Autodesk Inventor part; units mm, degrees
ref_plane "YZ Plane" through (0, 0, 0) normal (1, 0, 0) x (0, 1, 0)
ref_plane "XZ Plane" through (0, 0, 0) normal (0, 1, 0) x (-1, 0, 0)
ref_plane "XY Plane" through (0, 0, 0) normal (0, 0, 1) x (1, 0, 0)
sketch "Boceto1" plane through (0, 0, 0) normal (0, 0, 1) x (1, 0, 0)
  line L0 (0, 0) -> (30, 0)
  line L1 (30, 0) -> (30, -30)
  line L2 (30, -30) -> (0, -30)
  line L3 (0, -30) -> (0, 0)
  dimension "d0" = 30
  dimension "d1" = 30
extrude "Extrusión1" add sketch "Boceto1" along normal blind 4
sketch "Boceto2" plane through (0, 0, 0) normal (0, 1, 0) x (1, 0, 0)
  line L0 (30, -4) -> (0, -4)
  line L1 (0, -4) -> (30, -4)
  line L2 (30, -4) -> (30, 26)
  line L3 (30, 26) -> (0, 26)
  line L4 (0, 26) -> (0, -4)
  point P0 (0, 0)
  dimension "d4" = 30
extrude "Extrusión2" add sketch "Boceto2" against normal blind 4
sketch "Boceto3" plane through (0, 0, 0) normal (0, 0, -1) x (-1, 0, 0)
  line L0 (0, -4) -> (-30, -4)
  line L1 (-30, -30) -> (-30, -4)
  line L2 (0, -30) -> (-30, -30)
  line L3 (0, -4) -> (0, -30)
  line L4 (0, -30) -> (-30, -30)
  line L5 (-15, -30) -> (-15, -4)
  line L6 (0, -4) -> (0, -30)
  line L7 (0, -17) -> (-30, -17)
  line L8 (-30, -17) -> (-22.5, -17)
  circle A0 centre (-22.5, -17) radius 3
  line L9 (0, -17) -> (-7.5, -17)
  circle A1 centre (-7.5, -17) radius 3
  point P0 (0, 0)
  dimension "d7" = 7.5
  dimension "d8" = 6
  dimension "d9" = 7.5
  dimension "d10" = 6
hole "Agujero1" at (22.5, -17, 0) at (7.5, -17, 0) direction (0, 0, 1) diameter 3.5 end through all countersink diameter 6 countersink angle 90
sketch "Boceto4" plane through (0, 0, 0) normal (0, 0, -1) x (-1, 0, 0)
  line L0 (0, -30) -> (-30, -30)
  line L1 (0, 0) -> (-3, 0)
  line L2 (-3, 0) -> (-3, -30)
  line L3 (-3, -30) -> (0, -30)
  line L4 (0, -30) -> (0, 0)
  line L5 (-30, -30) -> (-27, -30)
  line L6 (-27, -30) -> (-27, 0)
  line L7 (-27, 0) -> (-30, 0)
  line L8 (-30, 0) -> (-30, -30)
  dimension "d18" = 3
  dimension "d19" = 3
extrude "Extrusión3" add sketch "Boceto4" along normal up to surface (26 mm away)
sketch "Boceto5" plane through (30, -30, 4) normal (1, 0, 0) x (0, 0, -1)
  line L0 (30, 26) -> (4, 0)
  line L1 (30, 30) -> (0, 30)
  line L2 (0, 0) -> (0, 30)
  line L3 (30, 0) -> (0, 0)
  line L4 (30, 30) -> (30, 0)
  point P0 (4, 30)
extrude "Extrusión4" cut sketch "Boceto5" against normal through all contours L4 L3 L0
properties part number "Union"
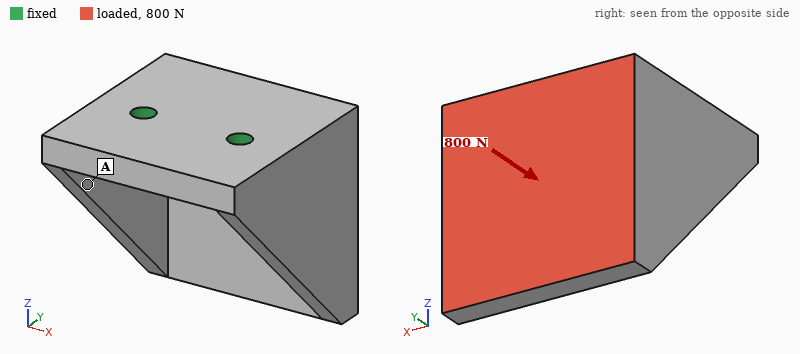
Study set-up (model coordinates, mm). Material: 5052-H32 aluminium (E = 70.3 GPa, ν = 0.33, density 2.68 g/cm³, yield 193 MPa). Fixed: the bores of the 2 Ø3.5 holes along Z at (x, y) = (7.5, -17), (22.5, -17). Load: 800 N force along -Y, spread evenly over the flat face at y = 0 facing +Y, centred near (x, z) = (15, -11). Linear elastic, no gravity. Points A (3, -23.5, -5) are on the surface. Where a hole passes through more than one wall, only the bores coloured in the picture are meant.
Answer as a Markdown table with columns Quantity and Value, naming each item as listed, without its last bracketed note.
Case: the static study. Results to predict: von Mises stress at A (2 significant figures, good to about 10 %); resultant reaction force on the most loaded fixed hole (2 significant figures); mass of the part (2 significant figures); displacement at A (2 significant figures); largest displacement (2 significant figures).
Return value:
| Quantity | Value |
|---|---|
| von Mises stress at A | 25 MPa |
| resultant reaction force on the most loaded fixed hole | 400 N |
| mass of the part | 23 g |
| displacement at A | 0.038 mm |
| largest displacement | 0.14 mm |
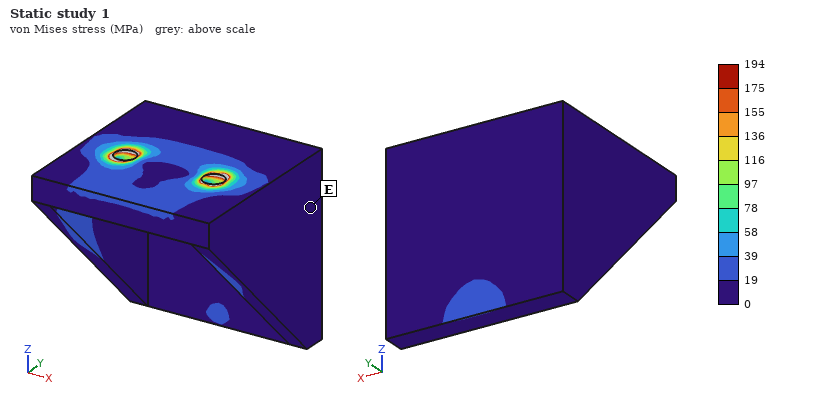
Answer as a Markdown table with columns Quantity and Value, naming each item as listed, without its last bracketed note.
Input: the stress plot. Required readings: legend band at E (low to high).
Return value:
| Quantity | Value |
|---|---|
| legend band at E | 0 to 19 MPa |
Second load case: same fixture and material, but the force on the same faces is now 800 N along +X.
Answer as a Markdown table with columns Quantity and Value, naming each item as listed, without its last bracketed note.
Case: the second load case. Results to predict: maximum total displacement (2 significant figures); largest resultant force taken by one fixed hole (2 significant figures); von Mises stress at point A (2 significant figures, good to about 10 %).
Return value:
| Quantity | Value |
|---|---|
| maximum total displacement | 80 µm |
| largest resultant force taken by one fixed hole | 1.0 kN |
| von Mises stress at point A | 24 MPa |
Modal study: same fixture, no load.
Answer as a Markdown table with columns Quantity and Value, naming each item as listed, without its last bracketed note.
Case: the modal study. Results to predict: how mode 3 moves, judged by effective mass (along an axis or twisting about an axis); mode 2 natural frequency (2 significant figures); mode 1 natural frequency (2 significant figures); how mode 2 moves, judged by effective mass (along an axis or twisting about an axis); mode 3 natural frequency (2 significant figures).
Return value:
| Quantity | Value |
|---|---|
| how mode 3 moves, judged by effective mass | along X |
| mode 2 natural frequency | 4600 Hz |
| mode 1 natural frequency | 3400 Hz |
| how mode 2 moves, judged by effective mass | along X |
| mode 3 natural frequency | 12 kHz |
